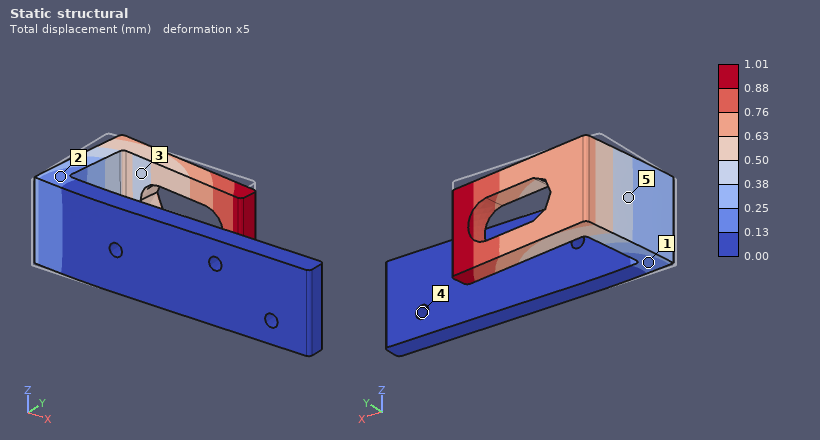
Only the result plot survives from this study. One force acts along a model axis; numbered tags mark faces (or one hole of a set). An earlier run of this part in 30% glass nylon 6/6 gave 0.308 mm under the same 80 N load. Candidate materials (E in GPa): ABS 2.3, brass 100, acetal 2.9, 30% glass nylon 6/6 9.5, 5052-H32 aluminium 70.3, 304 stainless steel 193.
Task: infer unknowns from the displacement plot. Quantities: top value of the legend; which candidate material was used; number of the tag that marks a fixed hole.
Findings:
1.01 mm
acetal
4
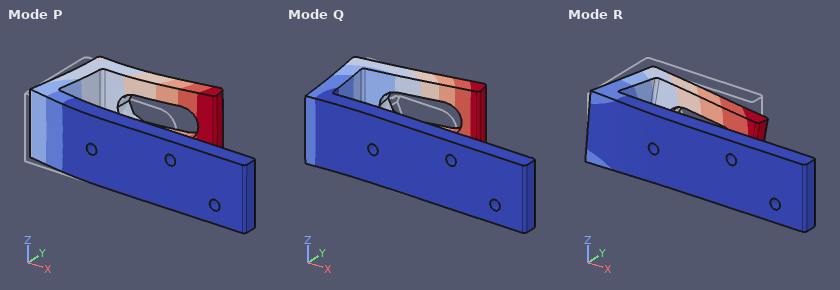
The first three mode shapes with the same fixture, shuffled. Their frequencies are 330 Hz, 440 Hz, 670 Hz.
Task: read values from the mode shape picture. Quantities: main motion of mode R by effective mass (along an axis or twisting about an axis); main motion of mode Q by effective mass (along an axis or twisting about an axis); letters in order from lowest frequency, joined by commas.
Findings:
along Z
along X
Q, R, P
